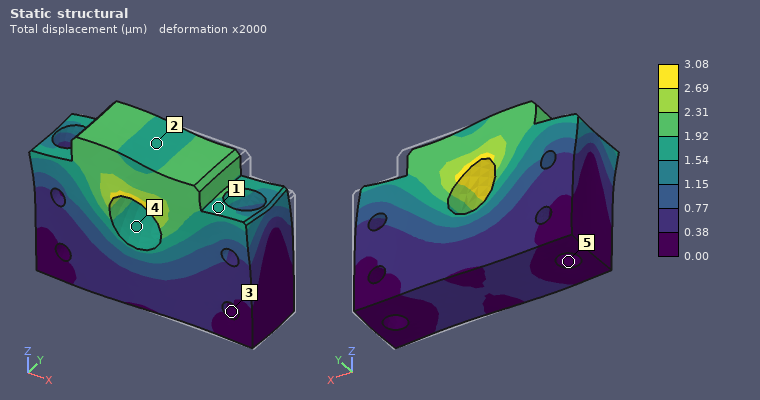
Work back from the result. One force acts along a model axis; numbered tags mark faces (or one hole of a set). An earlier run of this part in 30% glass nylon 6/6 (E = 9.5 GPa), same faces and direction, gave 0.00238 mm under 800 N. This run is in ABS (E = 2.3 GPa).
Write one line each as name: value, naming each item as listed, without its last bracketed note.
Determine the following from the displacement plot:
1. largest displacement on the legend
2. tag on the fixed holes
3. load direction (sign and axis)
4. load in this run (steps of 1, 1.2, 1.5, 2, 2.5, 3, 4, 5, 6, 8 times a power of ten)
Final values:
largest displacement on the legend: 3.08 µm
tag on the fixed holes: 5
load direction: -X
load in this run: 250 N
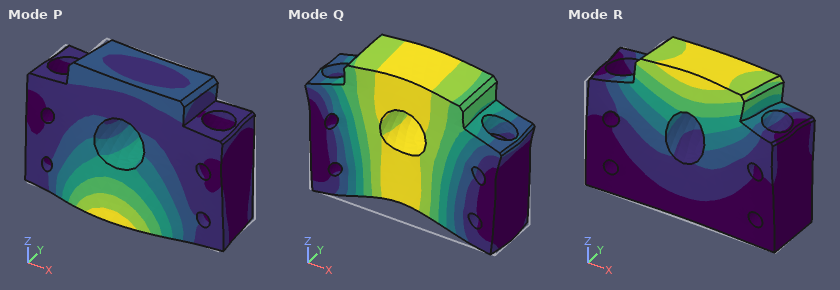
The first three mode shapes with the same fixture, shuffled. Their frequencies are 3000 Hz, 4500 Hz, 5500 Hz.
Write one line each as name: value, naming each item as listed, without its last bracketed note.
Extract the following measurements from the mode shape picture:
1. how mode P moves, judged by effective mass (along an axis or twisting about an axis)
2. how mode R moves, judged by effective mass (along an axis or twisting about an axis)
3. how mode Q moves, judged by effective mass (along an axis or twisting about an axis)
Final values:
how mode P moves, judged by effective mass: along Y
how mode R moves, judged by effective mass: along Y
how mode Q moves, judged by effective mass: along Z
